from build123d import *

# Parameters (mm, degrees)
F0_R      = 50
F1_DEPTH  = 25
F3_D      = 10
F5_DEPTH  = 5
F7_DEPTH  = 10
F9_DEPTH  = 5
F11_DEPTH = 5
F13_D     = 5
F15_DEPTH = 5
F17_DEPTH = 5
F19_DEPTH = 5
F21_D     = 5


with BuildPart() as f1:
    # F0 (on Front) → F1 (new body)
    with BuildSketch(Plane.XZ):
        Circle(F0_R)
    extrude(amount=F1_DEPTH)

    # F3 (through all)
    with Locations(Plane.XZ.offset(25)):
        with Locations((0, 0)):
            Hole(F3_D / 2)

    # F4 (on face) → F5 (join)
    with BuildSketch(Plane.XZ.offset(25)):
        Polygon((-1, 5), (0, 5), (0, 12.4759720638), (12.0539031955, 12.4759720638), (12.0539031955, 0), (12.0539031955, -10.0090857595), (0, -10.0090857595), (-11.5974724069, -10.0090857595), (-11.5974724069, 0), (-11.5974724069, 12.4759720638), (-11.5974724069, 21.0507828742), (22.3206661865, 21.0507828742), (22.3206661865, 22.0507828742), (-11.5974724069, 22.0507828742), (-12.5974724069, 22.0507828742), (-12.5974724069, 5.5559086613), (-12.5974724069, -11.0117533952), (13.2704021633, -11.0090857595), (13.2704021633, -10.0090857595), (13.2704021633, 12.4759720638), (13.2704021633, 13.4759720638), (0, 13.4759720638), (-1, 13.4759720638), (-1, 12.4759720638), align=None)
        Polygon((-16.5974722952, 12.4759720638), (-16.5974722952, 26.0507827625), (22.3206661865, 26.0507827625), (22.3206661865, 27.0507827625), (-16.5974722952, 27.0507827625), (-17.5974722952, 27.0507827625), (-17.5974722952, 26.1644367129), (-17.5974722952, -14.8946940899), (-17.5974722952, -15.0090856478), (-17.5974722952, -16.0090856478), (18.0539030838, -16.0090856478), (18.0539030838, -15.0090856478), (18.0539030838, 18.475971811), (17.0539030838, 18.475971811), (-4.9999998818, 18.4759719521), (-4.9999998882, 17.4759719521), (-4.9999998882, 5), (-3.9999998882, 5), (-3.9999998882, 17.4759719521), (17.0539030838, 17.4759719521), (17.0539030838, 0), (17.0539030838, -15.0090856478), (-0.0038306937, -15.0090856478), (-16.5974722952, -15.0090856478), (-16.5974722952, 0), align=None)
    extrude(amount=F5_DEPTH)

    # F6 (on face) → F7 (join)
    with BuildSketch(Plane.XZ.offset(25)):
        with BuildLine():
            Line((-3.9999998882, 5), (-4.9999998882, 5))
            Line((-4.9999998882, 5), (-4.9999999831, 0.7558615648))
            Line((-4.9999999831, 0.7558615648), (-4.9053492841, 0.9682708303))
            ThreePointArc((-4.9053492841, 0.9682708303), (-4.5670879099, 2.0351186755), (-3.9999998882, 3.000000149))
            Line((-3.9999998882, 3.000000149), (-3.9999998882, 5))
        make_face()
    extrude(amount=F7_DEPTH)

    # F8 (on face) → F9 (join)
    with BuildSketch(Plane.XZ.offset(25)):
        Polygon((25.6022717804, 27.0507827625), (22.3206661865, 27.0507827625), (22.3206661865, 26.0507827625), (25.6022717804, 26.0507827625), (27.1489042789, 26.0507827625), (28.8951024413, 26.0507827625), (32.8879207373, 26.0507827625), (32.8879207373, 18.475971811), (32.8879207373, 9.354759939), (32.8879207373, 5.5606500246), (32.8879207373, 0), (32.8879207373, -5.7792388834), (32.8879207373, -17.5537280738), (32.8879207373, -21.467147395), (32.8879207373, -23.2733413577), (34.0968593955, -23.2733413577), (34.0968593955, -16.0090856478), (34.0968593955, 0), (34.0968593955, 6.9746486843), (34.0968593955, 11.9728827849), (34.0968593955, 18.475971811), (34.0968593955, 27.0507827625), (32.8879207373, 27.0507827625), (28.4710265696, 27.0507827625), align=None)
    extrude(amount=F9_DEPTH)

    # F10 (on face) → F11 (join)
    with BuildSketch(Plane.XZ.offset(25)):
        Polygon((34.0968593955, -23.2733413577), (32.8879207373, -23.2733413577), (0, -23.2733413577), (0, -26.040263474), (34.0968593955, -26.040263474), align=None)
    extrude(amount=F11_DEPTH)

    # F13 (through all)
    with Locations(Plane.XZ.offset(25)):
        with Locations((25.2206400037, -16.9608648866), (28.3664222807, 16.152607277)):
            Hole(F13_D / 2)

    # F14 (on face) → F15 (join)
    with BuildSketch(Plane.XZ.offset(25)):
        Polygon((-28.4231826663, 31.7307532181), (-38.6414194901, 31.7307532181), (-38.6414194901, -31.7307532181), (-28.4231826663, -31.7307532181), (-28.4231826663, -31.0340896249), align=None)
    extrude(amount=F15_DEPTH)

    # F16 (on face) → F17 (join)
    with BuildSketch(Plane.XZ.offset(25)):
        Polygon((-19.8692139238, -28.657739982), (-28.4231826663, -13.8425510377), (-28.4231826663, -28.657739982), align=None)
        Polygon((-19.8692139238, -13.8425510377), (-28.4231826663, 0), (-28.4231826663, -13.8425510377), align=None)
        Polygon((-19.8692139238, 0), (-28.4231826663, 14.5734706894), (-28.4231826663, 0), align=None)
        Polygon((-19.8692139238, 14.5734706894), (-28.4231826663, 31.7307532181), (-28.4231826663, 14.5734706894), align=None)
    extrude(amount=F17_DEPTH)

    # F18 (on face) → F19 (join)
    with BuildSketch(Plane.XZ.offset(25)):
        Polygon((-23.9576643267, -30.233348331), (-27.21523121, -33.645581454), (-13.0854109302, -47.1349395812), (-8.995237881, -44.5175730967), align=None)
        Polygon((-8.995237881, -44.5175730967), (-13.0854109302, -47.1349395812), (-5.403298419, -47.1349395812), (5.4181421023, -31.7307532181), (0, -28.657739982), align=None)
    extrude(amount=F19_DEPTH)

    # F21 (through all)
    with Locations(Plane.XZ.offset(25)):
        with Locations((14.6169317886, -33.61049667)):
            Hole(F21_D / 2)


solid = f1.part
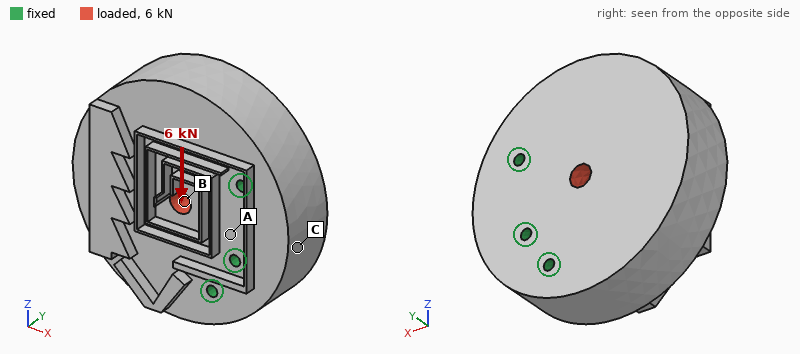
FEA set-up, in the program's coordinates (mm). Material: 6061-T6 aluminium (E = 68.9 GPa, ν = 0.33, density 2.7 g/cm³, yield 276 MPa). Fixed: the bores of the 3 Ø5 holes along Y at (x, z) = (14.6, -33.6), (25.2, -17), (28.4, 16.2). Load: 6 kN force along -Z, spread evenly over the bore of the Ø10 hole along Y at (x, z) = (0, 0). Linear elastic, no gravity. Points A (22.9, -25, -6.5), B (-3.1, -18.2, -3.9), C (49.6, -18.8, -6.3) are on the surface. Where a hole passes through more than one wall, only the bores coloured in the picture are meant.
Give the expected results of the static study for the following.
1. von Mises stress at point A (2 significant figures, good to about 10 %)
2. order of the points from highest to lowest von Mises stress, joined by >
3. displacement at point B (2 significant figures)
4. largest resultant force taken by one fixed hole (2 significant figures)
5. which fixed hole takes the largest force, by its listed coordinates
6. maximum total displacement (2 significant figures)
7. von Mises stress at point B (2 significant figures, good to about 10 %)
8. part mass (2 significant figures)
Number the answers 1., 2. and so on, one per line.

1. 3.8 MPa
2. B > A > C
3. 4.8 µm
4. 3.5 kN
5. (14.6, -33.6)
6. 6.1 µm
7. 10 MPa
8. 540 g
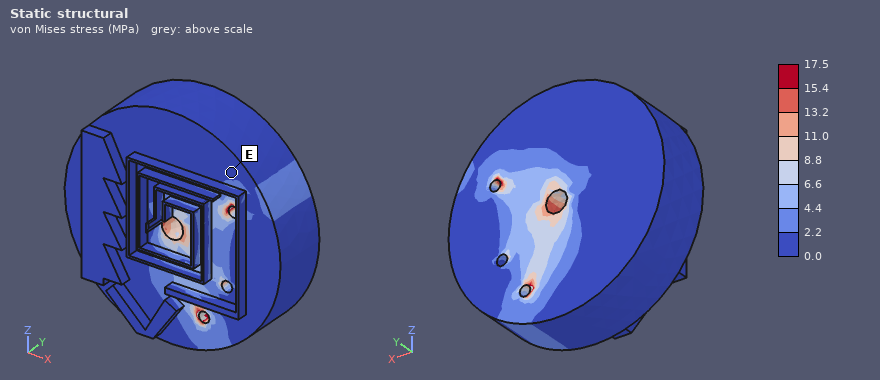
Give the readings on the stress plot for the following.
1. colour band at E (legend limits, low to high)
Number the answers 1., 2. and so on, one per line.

1. 0.0 to 2.2 MPa
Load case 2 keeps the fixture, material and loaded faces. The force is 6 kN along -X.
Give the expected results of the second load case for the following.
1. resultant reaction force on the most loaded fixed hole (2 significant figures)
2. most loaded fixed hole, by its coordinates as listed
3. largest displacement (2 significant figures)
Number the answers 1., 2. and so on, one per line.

1. 3.4 kN
2. (28.4, 16.2)
3. 3.4 µm
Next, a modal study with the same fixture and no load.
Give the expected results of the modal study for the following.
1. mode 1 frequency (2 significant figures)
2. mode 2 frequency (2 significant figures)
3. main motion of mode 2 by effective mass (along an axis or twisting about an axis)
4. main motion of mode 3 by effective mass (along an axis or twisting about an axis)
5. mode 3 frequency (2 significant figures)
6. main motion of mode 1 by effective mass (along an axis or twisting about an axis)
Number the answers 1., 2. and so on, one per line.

1. 3500 Hz
2. 6600 Hz
3. along Z
4. twisting about X
5. 7200 Hz
6. along Y
